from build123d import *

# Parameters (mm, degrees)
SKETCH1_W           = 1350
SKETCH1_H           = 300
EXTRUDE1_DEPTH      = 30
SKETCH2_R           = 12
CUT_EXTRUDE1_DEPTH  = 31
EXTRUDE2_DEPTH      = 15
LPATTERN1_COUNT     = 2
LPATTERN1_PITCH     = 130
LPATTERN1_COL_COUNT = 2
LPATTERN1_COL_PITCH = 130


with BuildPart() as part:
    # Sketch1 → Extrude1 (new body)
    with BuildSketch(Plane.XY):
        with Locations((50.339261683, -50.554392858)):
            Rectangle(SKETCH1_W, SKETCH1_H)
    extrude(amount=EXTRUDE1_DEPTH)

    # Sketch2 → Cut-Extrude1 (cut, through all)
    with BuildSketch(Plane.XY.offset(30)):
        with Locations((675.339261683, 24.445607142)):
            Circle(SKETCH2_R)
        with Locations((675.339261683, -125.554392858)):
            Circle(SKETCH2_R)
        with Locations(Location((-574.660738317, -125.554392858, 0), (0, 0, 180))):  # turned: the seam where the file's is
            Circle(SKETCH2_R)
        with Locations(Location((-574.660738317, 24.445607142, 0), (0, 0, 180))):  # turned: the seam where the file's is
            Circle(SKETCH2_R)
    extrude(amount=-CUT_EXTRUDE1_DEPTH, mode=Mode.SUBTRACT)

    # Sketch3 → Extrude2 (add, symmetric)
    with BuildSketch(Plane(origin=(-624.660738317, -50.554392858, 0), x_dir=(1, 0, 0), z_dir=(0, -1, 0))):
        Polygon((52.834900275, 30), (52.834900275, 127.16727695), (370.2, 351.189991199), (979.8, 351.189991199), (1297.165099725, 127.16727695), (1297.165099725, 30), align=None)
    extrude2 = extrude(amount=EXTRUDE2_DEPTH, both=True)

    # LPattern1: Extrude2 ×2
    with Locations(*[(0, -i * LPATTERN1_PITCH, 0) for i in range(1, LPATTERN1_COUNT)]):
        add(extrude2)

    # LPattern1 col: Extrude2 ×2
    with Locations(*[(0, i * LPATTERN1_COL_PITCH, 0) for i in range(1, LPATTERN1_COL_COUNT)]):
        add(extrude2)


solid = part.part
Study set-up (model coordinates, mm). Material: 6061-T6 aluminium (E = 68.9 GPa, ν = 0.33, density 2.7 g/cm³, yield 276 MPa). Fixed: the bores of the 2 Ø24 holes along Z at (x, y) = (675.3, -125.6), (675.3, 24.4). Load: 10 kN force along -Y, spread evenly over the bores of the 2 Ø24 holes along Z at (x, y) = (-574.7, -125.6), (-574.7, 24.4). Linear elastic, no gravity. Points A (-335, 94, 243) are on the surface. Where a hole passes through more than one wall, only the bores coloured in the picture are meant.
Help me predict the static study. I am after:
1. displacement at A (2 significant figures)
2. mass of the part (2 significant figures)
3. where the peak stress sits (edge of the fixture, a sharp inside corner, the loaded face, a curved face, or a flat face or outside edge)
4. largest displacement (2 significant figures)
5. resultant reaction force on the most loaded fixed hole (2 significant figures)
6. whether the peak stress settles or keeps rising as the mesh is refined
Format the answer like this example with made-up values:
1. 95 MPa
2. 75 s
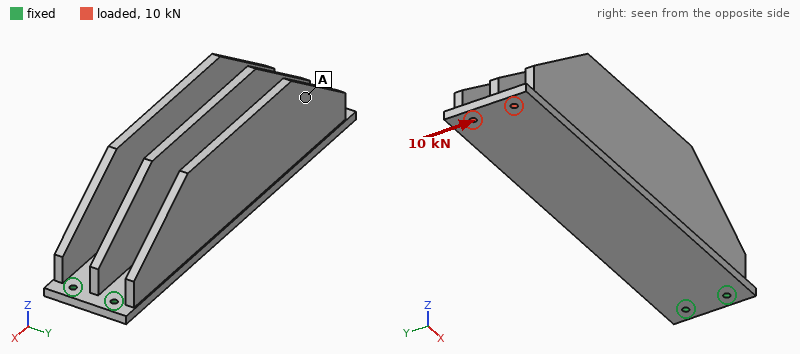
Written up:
1. 0.80 mm
2. 110 kg
3. edge of the fixture
4. 1.2 mm
5. 76 kN
6. keeps rising
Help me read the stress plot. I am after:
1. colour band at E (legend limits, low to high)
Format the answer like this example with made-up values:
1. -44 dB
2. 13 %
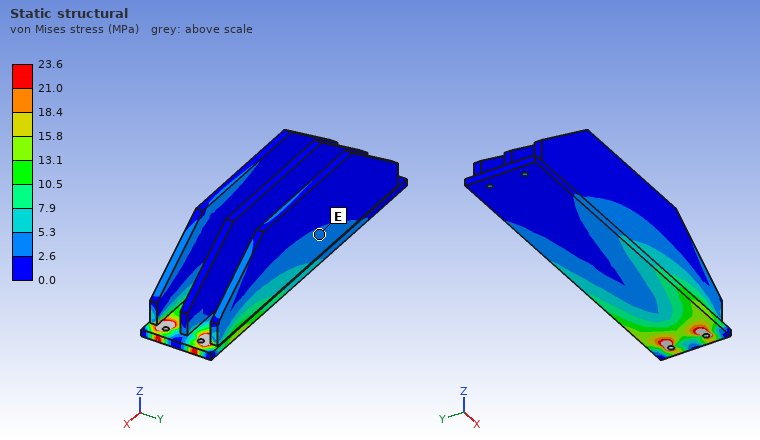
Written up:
1. 2.6 to 5.3 MPa
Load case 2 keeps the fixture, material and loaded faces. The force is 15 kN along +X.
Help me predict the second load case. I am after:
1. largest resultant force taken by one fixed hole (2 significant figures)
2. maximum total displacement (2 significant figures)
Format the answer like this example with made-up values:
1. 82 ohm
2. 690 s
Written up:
1. 7.5 kN
2. 87 µm
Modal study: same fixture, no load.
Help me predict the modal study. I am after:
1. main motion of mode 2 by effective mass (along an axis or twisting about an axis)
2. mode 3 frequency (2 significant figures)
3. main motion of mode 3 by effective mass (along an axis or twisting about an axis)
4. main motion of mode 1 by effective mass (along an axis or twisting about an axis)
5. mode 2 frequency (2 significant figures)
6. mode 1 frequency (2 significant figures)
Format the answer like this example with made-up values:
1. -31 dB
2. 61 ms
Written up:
1. along Y
2. 110 Hz
3. along Y
4. along Z
5. 56 Hz
6. 22 Hz
